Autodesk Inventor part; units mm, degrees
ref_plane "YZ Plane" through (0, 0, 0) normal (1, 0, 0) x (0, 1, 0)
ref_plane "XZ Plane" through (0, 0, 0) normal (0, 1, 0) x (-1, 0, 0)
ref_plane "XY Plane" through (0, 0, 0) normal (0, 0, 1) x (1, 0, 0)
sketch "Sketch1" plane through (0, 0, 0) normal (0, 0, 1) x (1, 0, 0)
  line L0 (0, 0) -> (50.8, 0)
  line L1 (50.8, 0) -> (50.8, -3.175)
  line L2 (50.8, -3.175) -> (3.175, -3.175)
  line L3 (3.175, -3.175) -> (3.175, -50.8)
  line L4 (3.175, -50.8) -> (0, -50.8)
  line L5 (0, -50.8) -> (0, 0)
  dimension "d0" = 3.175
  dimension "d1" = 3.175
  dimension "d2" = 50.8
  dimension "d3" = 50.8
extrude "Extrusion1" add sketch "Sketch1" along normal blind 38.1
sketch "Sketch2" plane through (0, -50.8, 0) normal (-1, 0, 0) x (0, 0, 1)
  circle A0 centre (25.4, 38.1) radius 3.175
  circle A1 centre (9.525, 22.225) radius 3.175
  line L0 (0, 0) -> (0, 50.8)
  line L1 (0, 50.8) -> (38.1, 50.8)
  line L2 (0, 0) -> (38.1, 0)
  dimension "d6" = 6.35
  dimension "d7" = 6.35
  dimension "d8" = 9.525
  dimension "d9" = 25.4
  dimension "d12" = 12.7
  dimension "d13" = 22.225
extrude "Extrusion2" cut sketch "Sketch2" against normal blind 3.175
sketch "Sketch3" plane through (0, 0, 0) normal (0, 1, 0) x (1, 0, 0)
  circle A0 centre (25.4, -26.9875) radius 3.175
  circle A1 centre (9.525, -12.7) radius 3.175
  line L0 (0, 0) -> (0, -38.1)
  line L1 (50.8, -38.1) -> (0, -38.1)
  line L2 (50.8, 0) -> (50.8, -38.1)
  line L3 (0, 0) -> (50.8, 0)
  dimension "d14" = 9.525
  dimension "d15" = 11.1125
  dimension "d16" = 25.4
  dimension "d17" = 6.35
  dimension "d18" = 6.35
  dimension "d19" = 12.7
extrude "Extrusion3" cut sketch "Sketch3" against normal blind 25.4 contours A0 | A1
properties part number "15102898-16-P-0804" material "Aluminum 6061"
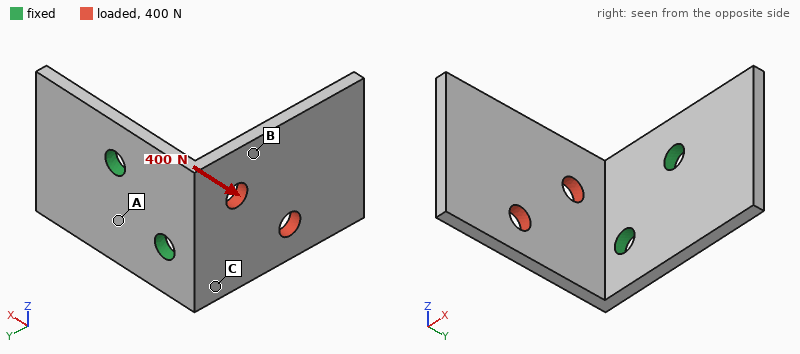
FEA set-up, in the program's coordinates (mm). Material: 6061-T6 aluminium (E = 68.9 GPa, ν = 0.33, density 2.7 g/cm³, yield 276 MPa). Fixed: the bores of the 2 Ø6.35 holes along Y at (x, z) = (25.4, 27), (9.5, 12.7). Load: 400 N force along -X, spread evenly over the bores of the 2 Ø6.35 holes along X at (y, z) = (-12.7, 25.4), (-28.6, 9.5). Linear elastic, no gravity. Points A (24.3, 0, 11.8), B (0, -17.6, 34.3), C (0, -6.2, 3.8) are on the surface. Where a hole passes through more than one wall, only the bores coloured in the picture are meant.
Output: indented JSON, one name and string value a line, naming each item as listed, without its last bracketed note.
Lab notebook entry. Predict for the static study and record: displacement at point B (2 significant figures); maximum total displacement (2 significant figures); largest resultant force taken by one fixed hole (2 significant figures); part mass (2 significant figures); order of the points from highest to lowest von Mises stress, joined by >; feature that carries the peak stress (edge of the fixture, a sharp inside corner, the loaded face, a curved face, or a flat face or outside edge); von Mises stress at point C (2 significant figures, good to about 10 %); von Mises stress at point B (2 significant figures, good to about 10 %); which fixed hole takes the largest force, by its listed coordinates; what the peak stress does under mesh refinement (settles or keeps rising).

{
  "displacement at point B": "0.21 mm",
  "maximum total displacement": "0.89 mm",
  "largest resultant force taken by one fixed hole": "300 N",
  "part mass": "31 g",
  "order of the points from highest to lowest von Mises stress, joined by >": "C > B > A",
  "feature that carries the peak stress": "edge of the fixture",
  "von Mises stress at point C": "99 MPa",
  "von Mises stress at point B": "36 MPa",
  "which fixed hole takes the largest force, by its listed coordinates": "(9.5, 12.7)",
  "what the peak stress does under mesh refinement": "keeps rising"
}
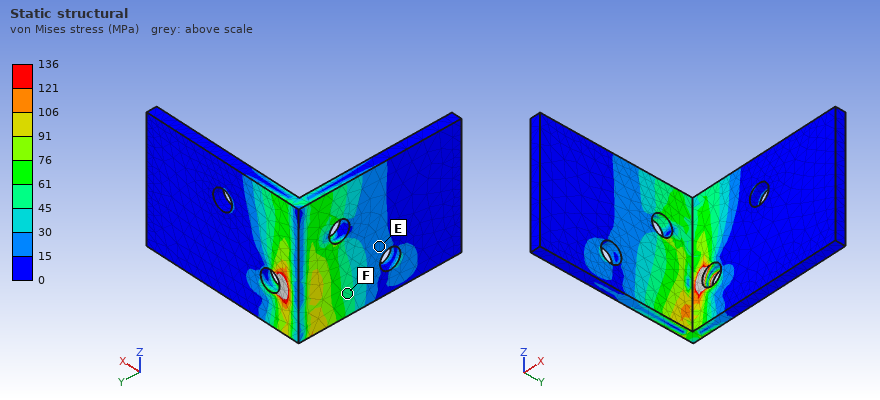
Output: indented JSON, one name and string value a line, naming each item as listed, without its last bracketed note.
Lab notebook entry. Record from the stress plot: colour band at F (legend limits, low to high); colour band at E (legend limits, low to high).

{
  "colour band at F": "45 to 61 MPa",
  "colour band at E": "15 to 30 MPa"
}
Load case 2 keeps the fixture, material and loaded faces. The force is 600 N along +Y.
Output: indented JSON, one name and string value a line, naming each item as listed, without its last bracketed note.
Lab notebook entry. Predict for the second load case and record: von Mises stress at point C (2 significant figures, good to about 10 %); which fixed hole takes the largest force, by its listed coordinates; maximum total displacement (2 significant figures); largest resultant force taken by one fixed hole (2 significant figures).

{
  "von Mises stress at point C": "11 MPa",
  "which fixed hole takes the largest force, by its listed coordinates": "(9.5, 12.7)",
  "maximum total displacement": "0.17 mm",
  "largest resultant force taken by one fixed hole": "590 N"
}
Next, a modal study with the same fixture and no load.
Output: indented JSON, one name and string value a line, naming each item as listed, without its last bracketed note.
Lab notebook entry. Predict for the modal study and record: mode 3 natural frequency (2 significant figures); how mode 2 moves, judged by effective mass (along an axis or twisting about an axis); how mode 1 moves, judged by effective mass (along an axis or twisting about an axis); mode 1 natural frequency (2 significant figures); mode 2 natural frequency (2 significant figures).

{
  "mode 3 natural frequency": "3000 Hz",
  "how mode 2 moves, judged by effective mass": "along Z",
  "how mode 1 moves, judged by effective mass": "along X",
  "mode 1 natural frequency": "860 Hz",
  "mode 2 natural frequency": "1800 Hz"
}
